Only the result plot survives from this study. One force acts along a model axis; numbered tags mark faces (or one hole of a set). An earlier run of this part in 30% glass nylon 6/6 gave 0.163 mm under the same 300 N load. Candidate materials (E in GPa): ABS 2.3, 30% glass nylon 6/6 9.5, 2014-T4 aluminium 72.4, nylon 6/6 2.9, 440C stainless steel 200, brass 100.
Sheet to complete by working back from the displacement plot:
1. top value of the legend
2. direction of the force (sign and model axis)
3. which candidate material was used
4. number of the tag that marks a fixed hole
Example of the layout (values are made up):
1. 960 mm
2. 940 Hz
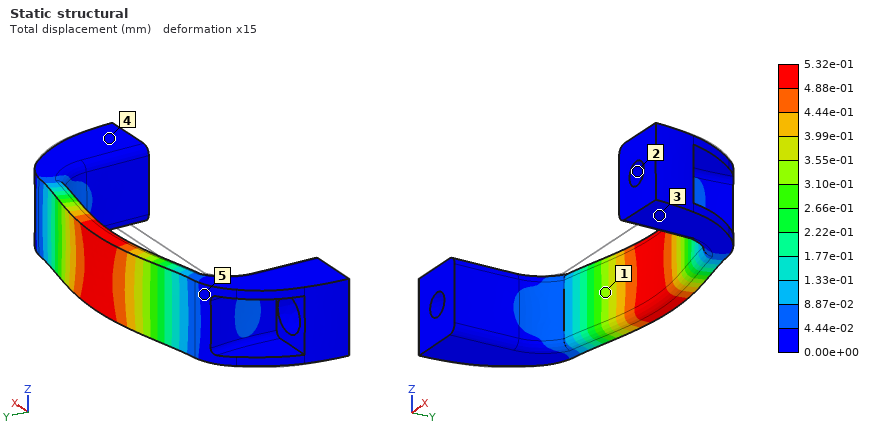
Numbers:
1. 5.32e-01 mm
2. +Y
3. nylon 6/6
4. 2
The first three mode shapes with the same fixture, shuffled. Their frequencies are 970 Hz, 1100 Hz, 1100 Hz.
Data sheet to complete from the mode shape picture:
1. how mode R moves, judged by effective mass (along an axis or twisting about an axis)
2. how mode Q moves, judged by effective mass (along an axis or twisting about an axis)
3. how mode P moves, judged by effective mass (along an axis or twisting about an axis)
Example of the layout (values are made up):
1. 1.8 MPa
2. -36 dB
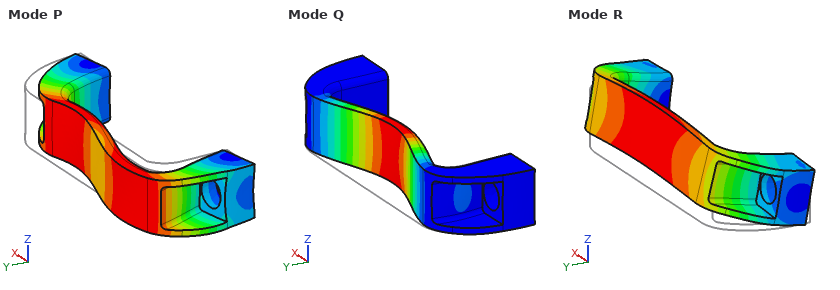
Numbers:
1. along Z
2. along Y
3. along X
